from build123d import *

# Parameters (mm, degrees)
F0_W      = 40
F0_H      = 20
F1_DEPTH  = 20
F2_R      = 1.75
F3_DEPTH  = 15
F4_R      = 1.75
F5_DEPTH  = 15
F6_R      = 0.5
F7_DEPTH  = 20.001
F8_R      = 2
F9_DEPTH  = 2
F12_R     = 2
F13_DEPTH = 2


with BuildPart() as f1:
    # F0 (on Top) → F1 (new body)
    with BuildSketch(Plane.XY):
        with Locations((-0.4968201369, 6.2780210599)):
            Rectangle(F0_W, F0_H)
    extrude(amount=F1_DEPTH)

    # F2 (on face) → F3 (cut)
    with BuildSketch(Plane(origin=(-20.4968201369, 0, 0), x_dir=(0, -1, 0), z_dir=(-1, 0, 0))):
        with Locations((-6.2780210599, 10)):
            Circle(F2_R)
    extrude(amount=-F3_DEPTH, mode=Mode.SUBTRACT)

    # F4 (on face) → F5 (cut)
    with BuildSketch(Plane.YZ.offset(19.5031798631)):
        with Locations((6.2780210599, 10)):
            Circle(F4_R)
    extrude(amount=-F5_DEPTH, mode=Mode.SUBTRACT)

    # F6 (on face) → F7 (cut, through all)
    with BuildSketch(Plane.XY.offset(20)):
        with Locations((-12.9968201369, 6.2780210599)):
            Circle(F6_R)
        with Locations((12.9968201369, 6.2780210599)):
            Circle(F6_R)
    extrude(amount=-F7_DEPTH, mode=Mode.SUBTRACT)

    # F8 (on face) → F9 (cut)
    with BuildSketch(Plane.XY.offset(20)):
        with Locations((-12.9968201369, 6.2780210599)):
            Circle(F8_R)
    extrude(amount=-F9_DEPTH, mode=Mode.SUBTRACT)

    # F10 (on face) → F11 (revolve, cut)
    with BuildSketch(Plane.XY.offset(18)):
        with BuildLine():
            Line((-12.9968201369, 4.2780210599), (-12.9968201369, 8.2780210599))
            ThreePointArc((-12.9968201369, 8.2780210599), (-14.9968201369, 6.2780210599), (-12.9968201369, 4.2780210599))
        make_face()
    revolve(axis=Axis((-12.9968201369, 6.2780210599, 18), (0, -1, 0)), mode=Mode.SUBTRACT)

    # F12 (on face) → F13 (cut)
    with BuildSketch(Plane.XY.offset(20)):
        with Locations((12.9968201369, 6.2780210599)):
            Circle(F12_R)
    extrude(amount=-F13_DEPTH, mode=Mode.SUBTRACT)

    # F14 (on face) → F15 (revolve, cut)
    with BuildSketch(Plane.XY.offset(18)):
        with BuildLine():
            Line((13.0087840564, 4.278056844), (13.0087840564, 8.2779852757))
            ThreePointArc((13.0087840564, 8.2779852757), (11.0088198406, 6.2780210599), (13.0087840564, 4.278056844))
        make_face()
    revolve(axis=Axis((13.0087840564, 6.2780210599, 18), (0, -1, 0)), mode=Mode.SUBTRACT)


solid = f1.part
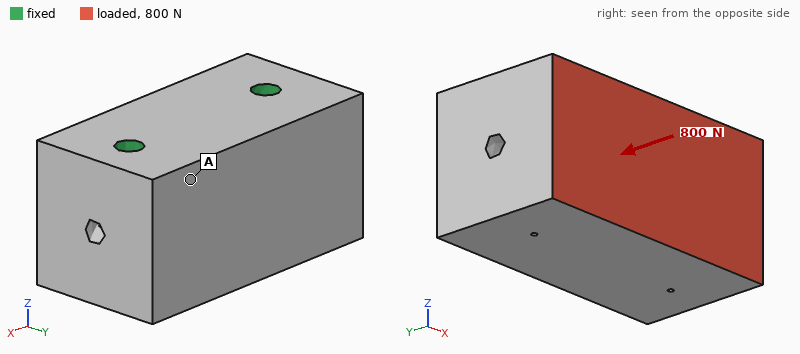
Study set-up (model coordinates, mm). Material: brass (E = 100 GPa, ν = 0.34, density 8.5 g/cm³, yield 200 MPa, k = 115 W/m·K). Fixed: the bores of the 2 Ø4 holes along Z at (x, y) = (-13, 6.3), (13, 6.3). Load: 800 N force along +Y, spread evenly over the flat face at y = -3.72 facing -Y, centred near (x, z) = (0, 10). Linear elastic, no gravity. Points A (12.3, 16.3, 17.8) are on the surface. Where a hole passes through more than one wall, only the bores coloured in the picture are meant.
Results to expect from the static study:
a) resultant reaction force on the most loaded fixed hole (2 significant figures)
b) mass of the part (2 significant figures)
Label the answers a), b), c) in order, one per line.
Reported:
a) 410 N
b) 130 g
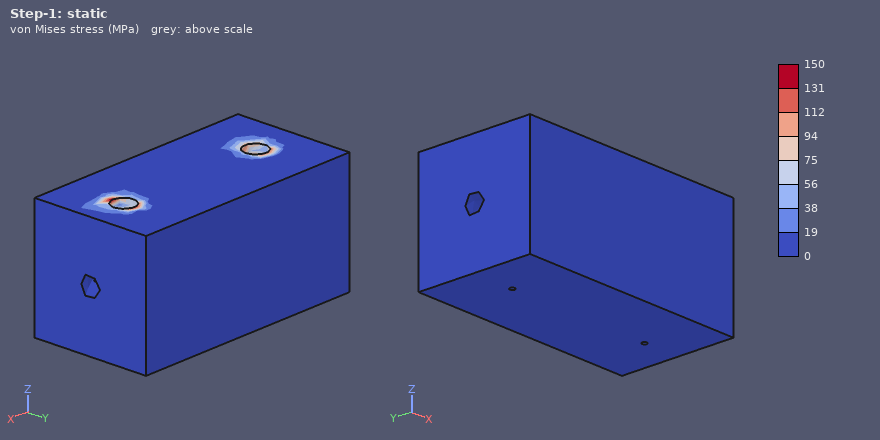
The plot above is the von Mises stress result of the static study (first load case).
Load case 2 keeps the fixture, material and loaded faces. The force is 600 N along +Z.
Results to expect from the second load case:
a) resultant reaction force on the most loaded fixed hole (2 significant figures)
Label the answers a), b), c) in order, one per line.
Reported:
a) 310 N
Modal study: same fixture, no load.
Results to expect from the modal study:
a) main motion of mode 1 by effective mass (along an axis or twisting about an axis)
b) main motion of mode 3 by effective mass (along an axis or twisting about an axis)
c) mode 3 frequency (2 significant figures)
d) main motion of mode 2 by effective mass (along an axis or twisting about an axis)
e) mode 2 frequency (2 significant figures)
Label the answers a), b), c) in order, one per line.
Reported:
a) along Y
b) twisting about Z
c) 13 kHz
d) along X
e) 11 kHz
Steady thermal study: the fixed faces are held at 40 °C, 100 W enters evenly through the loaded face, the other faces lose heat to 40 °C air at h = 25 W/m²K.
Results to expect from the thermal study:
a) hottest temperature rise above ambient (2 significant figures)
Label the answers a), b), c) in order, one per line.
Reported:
a) 40 K
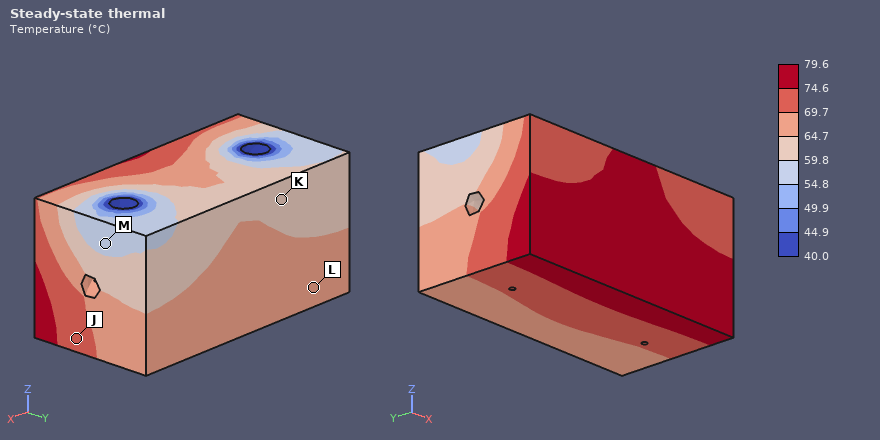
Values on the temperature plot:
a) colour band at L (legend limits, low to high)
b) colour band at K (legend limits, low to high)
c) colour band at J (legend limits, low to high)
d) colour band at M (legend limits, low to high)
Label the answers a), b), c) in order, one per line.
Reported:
a) 64.7 to 69.7 °C
b) 59.8 to 64.7 °C
c) 69.7 to 74.6 °C
d) 54.8 to 59.8 °C
